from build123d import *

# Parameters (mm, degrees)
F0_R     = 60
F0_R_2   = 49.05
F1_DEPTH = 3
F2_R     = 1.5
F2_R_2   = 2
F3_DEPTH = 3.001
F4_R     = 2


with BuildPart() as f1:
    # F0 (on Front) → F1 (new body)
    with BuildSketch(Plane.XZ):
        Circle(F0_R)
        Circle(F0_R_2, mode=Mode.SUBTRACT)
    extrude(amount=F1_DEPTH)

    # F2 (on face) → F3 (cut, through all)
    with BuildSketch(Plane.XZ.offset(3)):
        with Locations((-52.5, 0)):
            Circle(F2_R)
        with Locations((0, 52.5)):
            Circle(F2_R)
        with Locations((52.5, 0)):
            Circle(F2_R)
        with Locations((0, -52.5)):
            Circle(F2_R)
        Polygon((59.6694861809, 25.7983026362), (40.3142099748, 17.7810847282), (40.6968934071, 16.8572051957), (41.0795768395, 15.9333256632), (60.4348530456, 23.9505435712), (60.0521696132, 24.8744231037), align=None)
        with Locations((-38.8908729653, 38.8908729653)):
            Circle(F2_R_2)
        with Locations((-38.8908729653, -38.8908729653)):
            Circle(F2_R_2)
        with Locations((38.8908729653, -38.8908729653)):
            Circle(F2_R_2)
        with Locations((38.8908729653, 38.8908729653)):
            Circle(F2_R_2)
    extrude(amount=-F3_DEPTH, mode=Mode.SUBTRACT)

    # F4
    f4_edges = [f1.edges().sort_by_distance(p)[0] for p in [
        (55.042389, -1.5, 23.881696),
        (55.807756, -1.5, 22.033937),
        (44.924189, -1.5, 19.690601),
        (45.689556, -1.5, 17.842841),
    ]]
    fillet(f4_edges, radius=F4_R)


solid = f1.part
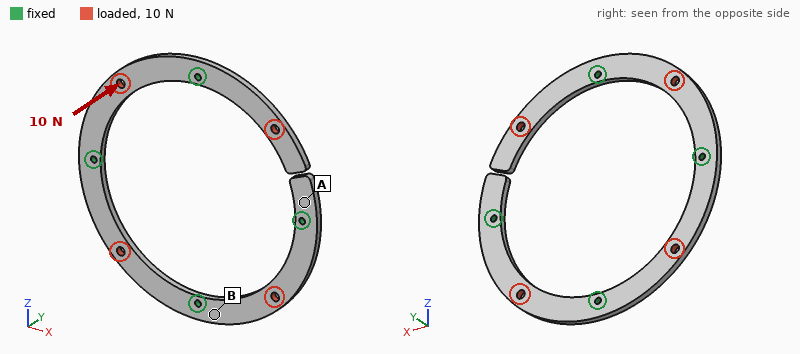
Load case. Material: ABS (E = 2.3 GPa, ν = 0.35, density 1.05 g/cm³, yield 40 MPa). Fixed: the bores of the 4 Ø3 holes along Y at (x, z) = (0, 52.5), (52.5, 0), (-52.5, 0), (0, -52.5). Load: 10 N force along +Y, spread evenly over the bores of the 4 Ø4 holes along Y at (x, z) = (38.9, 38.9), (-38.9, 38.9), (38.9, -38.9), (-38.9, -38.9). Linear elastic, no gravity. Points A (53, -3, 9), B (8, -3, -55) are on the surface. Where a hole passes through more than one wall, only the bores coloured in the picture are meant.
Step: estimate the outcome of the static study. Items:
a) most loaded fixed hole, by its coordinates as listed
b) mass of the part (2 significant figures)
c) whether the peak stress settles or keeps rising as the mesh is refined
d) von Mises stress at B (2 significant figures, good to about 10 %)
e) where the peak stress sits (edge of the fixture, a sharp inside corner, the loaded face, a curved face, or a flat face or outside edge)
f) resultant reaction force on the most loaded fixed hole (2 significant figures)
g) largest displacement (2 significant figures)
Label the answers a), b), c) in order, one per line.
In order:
a) (0, 52.5)
b) 11 g
c) keeps rising
d) 1.3 MPa
e) edge of the fixture
f) 3.7 N
g) 1.8 mm
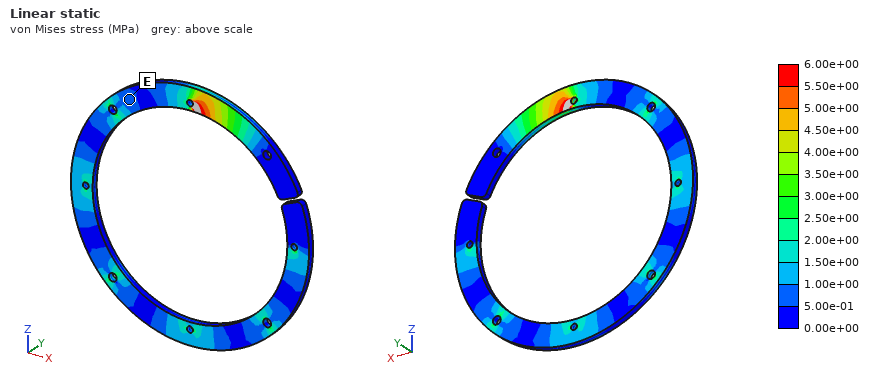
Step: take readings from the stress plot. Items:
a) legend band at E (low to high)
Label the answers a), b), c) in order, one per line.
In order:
a) 5.00e-01 to 1.00e+00 MPa
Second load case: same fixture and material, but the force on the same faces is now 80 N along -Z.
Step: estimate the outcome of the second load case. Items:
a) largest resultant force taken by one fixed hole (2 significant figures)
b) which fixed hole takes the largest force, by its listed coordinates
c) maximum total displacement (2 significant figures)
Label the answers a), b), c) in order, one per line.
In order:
a) 33 N
b) (0, 52.5)
c) 1.4 mm
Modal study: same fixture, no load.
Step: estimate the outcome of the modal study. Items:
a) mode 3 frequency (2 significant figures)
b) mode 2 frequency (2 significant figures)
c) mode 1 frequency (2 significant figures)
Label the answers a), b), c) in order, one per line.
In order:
a) 580 Hz
b) 570 Hz
c) 190 Hz
